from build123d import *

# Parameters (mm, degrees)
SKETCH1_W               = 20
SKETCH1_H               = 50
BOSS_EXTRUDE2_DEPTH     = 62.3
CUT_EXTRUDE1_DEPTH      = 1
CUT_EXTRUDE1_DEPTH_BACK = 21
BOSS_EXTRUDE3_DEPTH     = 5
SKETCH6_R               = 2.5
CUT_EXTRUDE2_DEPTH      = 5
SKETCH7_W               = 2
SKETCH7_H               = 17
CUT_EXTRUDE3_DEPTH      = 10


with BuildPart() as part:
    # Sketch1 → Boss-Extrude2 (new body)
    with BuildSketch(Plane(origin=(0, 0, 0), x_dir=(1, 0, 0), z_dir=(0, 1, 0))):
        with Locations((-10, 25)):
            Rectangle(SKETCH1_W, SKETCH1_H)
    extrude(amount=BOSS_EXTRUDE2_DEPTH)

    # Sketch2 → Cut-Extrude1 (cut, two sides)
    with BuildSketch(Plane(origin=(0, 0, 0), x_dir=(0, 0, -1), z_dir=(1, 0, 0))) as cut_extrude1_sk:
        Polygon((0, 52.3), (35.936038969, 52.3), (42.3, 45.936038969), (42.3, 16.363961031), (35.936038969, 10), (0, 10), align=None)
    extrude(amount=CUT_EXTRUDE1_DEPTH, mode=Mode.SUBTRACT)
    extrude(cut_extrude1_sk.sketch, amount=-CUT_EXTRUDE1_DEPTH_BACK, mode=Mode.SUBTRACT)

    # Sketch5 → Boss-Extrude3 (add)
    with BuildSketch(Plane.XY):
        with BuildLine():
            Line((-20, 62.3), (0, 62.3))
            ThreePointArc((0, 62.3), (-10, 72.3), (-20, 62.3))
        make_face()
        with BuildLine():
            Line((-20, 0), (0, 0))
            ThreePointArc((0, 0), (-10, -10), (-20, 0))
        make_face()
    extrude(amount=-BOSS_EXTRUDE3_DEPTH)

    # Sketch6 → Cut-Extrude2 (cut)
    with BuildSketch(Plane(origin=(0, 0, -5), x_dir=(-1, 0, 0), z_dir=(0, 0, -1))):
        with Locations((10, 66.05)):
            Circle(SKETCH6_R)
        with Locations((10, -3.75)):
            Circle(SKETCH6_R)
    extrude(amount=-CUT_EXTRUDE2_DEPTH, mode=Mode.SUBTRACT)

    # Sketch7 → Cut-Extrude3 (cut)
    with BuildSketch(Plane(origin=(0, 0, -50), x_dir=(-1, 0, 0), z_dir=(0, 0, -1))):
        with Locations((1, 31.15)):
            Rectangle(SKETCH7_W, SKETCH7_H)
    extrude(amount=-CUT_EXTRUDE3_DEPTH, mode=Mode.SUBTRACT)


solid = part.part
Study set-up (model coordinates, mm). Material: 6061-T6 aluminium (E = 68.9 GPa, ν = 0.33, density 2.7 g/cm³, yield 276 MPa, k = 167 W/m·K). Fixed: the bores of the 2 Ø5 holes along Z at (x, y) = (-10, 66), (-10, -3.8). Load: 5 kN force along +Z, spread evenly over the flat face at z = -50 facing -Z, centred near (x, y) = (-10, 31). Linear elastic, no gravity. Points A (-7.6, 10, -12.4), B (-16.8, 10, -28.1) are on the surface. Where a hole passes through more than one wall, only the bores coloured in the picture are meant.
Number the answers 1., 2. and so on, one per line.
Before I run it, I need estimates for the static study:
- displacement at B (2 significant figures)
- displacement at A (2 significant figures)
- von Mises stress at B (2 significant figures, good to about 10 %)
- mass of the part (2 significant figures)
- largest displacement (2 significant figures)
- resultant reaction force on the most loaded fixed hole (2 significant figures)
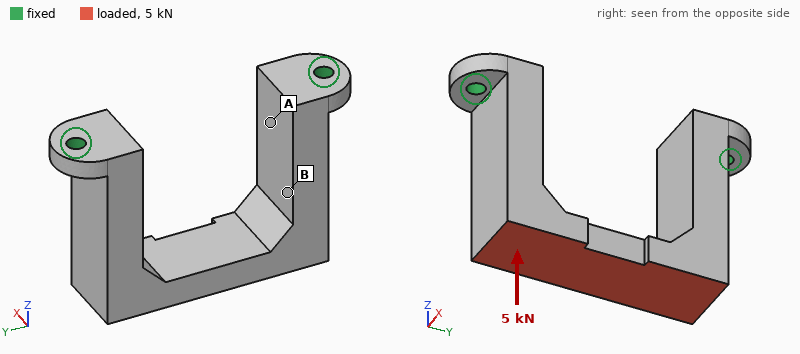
1. 17 µm
2. 11 µm
3. 30 MPa
4. 77 g
5. 48 µm
6. 2.6 kN
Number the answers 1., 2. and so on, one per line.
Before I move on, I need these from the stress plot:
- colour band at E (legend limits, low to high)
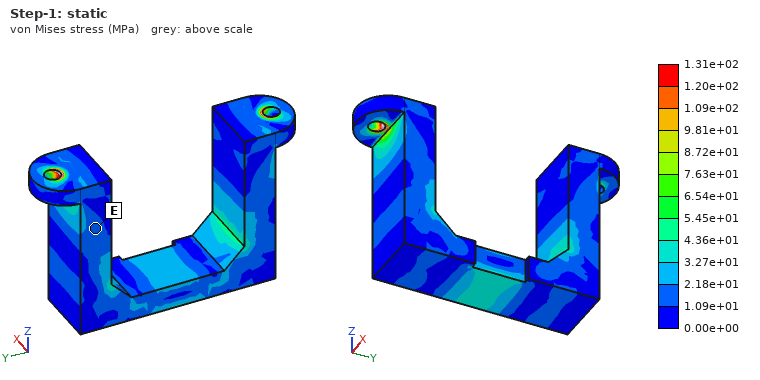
1. 1.09e+01 to 2.18e+01 MPa
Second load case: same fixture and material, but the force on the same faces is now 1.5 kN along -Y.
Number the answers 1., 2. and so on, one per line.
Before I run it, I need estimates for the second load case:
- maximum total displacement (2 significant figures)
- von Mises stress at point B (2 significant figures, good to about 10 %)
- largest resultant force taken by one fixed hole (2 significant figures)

1. 0.12 mm
2. 29 MPa
3. 1.2 kN
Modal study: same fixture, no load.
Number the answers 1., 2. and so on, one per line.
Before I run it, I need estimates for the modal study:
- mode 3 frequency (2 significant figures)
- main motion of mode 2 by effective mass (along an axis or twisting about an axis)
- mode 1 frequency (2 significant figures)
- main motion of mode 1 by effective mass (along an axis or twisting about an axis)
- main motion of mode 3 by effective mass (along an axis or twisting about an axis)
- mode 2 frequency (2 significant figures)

1. 3600 Hz
2. along Y
3. 1600 Hz
4. along X
5. twisting about Z
6. 2800 Hz
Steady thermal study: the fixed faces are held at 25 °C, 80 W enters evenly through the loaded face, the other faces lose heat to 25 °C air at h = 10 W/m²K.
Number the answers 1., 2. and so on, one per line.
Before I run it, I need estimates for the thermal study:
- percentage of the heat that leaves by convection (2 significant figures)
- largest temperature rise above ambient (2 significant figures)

1. 4.0 %
2. 73 K
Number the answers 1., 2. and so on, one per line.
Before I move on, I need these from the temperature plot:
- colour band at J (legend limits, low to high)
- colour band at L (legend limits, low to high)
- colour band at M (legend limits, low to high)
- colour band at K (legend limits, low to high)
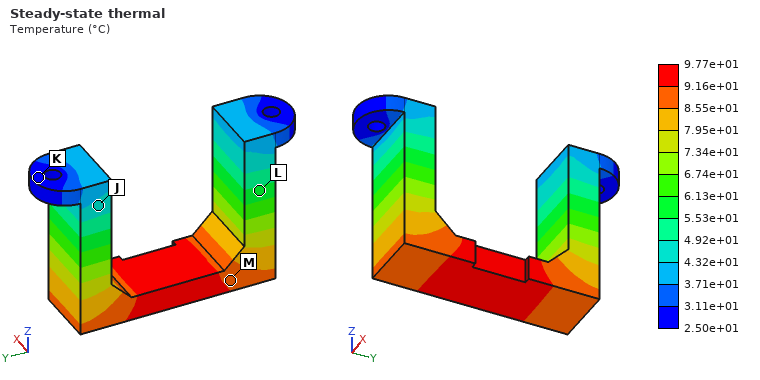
1. 4.32e+01 to 4.92e+01 °C
2. 5.53e+01 to 6.13e+01 °C
3. 8.55e+01 to 9.16e+01 °C
4. 2.50e+01 to 3.11e+01 °C
